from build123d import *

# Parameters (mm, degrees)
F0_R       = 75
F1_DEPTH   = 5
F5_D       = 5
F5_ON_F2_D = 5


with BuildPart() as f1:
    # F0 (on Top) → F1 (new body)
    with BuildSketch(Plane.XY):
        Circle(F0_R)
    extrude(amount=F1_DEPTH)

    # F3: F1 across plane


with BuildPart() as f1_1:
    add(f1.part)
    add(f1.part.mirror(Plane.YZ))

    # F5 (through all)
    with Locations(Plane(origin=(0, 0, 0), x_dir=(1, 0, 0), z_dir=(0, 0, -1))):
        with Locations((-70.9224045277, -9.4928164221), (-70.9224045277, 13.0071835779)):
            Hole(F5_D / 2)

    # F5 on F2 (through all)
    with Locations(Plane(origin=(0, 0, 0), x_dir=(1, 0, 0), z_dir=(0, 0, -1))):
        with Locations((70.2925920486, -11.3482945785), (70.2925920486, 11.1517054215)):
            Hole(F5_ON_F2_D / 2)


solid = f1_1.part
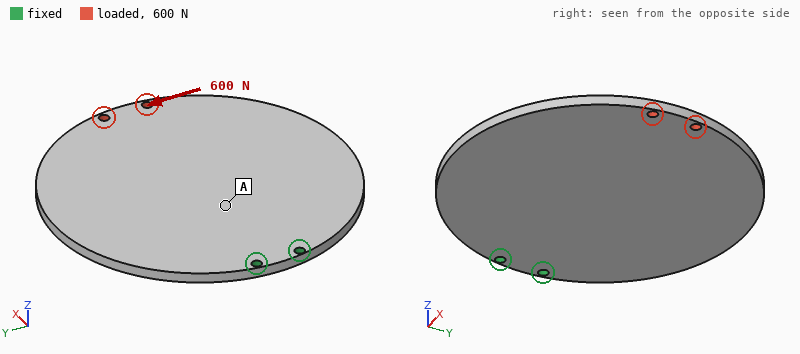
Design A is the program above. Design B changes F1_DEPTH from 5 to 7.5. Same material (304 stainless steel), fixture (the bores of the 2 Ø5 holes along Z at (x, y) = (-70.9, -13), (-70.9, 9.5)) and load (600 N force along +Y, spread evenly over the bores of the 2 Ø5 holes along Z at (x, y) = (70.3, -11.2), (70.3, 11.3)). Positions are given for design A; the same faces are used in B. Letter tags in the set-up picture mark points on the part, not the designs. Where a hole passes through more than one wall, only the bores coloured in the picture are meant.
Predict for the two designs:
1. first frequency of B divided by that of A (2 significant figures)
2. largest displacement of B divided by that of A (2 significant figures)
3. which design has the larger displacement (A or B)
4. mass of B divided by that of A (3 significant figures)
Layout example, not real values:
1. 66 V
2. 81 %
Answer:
1. 1.4
2. 0.67
3. A
4. 1.50
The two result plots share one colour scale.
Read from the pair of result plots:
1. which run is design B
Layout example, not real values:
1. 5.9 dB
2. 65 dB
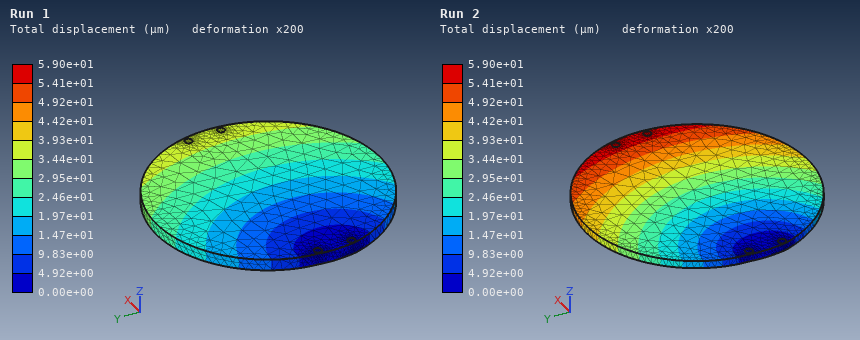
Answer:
1. Run 1
